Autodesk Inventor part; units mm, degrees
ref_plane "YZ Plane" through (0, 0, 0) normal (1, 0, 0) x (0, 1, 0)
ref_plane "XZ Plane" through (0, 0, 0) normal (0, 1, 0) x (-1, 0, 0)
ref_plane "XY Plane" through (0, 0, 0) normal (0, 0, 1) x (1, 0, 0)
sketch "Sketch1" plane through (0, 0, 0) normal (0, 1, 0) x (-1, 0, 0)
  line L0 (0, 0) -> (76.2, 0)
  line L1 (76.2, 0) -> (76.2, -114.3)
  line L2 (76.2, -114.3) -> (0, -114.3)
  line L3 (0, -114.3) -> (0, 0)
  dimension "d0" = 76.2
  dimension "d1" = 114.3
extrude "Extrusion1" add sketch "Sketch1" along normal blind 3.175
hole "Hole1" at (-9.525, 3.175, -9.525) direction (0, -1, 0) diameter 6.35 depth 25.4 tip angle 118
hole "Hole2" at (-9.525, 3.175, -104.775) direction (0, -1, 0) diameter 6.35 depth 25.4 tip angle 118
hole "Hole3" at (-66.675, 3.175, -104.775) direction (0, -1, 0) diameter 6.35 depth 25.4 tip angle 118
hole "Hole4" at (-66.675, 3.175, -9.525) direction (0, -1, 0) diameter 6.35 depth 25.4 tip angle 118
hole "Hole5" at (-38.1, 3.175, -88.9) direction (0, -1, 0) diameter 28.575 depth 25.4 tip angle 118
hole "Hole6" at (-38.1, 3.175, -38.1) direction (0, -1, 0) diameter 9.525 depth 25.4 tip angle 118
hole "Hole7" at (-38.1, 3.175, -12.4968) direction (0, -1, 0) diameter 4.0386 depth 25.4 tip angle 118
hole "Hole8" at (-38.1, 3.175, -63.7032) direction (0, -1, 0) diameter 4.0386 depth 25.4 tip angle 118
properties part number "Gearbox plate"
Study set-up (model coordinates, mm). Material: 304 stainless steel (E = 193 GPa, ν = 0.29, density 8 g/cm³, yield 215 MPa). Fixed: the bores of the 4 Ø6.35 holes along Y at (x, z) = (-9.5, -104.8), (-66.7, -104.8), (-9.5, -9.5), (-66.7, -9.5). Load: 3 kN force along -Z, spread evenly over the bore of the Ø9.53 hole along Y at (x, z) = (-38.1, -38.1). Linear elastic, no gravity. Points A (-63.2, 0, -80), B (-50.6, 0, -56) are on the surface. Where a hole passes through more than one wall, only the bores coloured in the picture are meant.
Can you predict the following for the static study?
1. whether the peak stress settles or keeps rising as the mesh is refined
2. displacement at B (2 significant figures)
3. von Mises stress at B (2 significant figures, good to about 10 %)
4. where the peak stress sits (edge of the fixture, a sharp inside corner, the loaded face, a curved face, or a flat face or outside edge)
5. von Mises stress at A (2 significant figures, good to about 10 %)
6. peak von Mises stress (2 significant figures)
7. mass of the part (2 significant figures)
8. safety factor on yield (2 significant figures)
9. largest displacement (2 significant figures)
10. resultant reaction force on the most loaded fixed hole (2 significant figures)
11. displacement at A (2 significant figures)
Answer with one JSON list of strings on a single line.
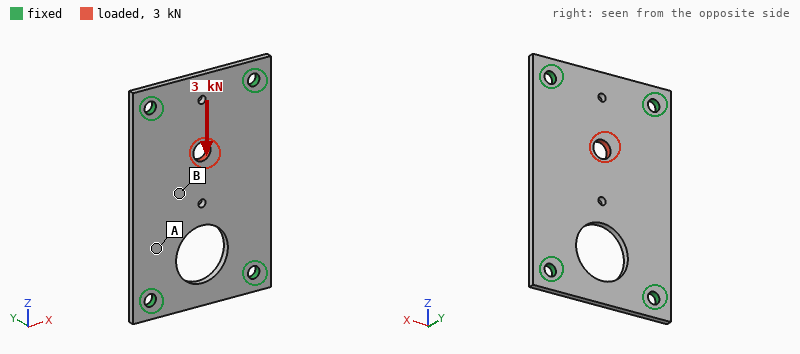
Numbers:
["settles", "2.3 µm", "12 MPa", "the loaded face", "6.0 MPa", "55 MPa", "200 g", "3.9", "4.3 µm", "1.1 kN", "1.1 µm"]
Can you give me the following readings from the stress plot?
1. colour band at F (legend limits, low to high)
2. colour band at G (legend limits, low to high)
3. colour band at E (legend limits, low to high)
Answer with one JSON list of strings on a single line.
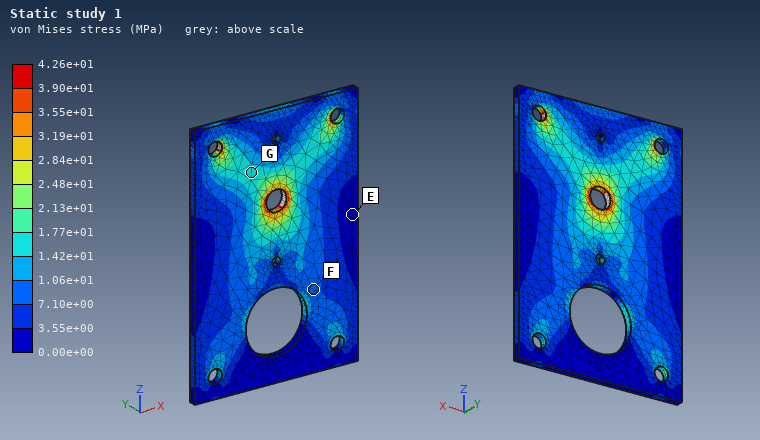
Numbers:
["7.10e+00 to 1.06e+01 MPa", "1.42e+01 to 1.77e+01 MPa", "0.00e+00 to 3.55e+00 MPa"]
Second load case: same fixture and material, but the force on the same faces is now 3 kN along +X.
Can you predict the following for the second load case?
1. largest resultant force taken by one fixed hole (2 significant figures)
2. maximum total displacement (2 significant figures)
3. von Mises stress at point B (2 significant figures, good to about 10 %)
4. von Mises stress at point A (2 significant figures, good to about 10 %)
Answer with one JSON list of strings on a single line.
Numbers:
["1.4 kN", "6.6 µm", "8.1 MPa", "7.4 MPa"]
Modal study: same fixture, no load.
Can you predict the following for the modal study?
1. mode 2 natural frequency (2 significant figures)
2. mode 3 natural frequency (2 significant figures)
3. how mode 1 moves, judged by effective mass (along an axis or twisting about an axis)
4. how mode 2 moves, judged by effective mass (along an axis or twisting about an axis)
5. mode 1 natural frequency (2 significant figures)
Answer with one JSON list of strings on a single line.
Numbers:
["2300 Hz", "3900 Hz", "along Y", "twisting about Z", "1700 Hz"]
